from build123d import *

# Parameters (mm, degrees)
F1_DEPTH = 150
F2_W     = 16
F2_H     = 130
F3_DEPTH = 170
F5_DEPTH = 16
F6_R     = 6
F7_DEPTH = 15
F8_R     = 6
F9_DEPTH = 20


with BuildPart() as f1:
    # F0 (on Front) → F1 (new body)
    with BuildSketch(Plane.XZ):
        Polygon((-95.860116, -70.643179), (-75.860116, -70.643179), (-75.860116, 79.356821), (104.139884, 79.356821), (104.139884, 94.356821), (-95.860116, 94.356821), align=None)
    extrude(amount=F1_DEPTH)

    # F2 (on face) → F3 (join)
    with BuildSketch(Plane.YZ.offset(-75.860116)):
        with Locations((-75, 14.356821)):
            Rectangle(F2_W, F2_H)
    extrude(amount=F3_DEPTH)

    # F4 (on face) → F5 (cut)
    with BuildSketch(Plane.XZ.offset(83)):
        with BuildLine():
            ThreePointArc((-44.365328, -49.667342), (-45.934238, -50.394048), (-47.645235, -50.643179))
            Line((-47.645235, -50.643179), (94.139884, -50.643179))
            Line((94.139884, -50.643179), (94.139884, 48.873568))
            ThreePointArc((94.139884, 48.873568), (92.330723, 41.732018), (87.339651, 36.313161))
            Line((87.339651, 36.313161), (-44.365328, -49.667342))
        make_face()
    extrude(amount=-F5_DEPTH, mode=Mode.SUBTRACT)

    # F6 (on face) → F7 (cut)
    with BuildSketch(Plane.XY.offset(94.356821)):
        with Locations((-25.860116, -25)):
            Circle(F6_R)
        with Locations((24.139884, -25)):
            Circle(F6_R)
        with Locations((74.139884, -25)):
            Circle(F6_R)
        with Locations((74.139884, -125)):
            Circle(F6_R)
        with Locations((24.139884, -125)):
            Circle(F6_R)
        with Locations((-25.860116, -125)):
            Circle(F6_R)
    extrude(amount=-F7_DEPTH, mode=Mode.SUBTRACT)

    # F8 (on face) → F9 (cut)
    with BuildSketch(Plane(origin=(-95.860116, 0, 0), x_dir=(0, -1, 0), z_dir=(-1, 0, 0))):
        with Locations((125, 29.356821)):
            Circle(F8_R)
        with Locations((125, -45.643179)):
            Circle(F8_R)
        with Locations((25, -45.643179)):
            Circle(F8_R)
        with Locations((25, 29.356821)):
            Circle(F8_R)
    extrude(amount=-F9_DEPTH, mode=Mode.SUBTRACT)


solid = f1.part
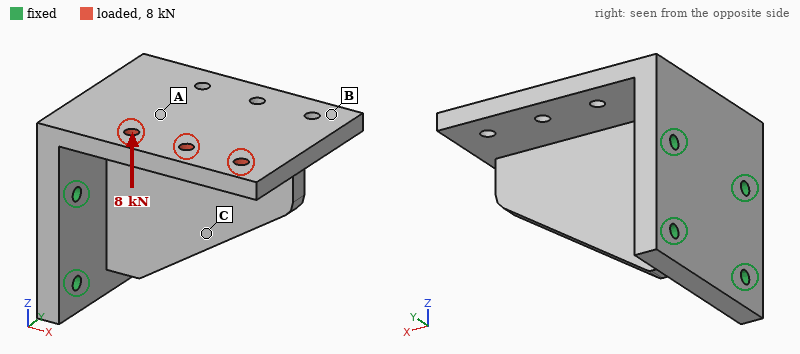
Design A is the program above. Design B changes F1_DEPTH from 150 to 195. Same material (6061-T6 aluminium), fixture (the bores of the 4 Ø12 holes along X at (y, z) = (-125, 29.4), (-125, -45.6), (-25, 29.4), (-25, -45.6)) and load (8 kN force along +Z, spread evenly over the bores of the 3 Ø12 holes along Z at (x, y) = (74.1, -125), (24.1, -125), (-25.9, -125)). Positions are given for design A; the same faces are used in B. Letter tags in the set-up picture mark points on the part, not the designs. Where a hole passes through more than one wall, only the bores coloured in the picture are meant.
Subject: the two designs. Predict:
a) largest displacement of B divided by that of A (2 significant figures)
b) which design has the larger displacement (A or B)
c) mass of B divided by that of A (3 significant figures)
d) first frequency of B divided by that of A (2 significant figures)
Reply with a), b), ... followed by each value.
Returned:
a) 1.1
b) B
c) 1.24
d) 0.91
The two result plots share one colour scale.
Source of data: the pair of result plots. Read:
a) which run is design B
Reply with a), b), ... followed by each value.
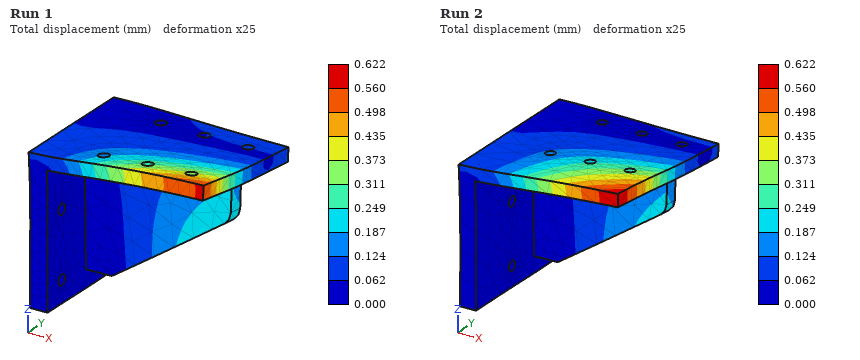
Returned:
a) Run 2
